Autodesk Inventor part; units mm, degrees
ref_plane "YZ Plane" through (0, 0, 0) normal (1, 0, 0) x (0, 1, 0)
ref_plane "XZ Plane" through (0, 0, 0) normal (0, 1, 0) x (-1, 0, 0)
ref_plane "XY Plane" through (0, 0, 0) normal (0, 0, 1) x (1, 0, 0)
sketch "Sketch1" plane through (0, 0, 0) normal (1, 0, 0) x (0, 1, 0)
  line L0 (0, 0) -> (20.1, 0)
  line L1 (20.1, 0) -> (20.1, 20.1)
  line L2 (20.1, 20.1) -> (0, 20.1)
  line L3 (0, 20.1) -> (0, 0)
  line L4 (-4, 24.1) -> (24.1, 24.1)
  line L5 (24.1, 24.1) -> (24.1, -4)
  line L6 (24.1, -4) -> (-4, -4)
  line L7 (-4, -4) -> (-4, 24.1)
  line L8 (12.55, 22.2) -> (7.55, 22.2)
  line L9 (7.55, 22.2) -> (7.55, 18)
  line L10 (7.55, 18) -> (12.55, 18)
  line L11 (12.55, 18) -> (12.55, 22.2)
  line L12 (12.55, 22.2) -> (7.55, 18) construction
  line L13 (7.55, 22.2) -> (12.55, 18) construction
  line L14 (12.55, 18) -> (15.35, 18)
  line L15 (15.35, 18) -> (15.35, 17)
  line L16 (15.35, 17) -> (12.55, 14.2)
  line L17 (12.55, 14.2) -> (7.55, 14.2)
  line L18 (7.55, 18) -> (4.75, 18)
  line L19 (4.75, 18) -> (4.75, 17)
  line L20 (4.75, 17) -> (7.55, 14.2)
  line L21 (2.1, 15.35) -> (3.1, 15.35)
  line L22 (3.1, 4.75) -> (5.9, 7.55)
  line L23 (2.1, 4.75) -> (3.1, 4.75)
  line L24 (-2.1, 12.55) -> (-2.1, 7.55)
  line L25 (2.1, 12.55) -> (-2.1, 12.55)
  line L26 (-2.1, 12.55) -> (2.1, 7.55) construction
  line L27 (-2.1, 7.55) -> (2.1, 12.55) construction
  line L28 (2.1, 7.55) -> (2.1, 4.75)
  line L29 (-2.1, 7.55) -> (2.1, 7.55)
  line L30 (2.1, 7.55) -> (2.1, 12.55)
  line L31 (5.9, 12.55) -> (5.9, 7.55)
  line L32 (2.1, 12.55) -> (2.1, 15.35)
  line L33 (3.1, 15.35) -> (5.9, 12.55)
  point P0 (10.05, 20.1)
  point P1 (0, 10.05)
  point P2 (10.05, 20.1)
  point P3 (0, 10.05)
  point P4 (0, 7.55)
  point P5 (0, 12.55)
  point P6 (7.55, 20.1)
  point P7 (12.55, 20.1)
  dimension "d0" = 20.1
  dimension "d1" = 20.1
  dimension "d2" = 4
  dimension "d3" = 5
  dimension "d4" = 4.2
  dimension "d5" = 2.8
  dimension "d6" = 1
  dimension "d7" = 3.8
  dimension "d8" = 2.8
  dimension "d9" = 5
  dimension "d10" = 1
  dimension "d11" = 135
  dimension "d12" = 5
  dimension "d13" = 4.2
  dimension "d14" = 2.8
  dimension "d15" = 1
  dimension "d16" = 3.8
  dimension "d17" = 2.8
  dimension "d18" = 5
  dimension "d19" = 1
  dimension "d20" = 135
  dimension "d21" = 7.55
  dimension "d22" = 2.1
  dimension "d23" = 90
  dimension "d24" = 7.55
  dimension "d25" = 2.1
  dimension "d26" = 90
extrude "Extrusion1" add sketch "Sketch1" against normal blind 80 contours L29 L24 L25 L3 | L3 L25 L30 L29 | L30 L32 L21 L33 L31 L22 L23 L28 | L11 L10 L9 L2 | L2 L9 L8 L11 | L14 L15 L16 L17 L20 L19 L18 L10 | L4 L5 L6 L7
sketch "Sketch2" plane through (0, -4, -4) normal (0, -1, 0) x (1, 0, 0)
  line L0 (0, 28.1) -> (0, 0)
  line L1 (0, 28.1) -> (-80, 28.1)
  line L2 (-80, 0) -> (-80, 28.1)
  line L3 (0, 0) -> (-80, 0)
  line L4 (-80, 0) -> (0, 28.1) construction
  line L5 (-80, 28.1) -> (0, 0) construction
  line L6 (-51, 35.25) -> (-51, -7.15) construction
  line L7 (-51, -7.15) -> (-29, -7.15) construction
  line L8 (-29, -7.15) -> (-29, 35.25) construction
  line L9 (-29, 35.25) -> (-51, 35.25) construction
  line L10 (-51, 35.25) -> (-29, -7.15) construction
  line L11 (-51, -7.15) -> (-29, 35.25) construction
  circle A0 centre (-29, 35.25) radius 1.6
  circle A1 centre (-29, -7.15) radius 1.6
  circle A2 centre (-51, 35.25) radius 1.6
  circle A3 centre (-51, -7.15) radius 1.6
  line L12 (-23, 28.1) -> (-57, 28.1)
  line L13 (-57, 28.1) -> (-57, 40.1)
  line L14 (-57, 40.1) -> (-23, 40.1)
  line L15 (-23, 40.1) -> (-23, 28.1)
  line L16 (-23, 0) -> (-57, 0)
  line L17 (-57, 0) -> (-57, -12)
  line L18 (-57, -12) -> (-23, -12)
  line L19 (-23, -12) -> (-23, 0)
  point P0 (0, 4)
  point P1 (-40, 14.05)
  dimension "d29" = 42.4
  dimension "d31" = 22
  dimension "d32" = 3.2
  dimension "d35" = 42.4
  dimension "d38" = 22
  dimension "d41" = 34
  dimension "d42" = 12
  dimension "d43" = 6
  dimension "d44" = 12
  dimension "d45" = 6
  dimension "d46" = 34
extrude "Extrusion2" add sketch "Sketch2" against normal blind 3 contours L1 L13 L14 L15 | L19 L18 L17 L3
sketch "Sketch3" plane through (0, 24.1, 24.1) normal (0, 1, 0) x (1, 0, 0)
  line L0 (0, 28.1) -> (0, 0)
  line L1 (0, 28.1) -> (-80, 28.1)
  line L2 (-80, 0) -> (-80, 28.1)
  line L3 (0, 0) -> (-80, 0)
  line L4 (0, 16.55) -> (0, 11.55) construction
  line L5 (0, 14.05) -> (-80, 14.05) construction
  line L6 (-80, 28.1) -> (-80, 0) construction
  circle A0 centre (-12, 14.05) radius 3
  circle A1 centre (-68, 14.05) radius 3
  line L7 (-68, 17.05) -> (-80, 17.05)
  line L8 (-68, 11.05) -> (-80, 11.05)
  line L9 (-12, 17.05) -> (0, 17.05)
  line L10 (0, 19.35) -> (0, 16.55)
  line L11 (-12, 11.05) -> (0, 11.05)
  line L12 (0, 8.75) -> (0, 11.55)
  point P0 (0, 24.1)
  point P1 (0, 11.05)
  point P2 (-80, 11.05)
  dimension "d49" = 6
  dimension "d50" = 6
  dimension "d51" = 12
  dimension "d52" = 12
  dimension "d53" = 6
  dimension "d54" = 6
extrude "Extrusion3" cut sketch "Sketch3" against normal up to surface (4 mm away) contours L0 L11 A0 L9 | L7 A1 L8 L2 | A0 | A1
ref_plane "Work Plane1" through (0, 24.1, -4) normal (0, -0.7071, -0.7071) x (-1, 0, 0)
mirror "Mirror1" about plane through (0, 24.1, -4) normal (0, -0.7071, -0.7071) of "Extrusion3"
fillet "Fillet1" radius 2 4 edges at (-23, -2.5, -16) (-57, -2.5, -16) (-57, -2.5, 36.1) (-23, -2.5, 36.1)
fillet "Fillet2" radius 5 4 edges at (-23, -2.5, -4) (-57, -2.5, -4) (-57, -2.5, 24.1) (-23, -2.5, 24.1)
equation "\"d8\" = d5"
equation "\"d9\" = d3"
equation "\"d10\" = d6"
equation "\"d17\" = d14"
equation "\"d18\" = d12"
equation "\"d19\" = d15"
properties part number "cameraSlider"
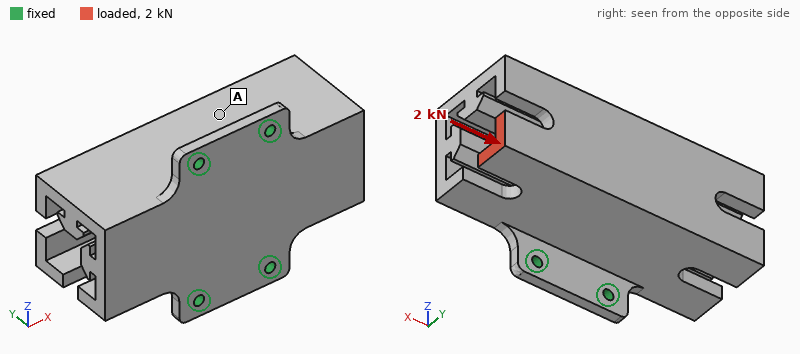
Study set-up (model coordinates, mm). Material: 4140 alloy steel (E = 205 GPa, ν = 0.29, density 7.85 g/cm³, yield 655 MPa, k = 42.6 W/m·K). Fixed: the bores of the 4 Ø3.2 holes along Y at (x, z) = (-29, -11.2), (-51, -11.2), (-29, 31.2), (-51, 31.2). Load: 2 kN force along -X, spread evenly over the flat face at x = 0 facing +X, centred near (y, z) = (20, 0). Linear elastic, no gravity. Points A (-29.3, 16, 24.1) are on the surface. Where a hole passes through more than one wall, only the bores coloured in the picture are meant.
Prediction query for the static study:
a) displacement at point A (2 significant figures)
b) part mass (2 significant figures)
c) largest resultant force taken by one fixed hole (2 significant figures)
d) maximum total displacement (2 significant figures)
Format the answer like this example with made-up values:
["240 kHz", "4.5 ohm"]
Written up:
["22 µm", "300 g", "1.2 kN", "60 µm"]
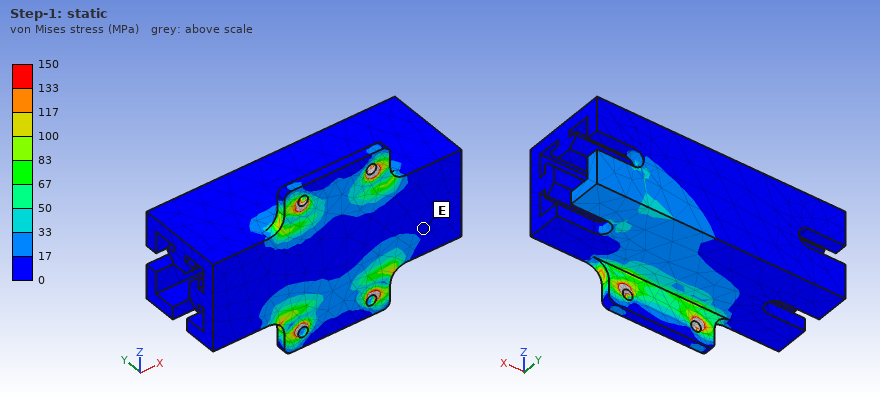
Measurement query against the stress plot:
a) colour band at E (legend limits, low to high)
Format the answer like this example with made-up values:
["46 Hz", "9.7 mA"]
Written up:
["0 to 17 MPa"]
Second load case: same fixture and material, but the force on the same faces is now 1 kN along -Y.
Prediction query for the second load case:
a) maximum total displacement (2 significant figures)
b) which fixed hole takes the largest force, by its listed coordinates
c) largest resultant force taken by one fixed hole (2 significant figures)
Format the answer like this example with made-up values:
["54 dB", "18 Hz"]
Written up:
["88 µm", "(-29, -11.2)", "1.3 kN"]
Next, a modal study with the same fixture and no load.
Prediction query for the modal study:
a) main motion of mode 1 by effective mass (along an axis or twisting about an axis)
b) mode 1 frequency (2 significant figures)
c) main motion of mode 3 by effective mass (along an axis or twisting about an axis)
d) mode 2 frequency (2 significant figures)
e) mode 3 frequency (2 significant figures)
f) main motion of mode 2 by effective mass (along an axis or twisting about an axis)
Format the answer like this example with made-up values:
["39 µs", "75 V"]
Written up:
["along X", "2300 Hz", "along Y", "3900 Hz", "4900 Hz", "along Z"]
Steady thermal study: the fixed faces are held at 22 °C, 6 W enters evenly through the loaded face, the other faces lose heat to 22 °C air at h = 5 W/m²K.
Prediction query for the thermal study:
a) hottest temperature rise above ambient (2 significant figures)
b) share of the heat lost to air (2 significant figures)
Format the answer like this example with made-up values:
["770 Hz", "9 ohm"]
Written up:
["56 K", "15 %"]
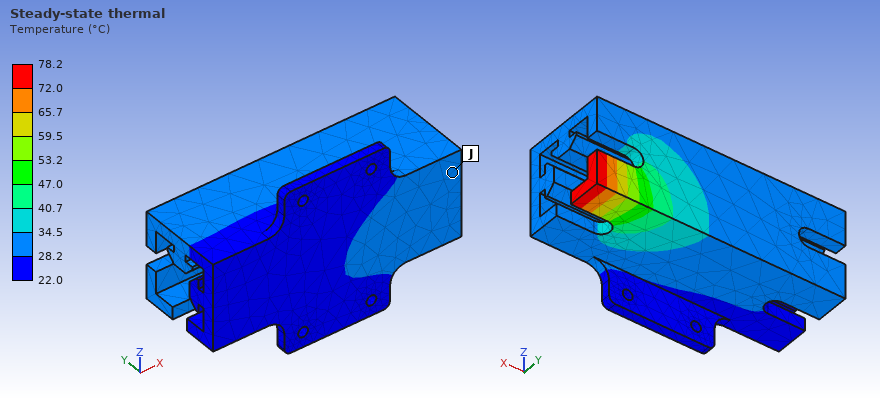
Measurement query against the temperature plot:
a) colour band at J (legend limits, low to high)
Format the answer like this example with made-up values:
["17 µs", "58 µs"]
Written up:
["28.2 to 34.5 °C"]
